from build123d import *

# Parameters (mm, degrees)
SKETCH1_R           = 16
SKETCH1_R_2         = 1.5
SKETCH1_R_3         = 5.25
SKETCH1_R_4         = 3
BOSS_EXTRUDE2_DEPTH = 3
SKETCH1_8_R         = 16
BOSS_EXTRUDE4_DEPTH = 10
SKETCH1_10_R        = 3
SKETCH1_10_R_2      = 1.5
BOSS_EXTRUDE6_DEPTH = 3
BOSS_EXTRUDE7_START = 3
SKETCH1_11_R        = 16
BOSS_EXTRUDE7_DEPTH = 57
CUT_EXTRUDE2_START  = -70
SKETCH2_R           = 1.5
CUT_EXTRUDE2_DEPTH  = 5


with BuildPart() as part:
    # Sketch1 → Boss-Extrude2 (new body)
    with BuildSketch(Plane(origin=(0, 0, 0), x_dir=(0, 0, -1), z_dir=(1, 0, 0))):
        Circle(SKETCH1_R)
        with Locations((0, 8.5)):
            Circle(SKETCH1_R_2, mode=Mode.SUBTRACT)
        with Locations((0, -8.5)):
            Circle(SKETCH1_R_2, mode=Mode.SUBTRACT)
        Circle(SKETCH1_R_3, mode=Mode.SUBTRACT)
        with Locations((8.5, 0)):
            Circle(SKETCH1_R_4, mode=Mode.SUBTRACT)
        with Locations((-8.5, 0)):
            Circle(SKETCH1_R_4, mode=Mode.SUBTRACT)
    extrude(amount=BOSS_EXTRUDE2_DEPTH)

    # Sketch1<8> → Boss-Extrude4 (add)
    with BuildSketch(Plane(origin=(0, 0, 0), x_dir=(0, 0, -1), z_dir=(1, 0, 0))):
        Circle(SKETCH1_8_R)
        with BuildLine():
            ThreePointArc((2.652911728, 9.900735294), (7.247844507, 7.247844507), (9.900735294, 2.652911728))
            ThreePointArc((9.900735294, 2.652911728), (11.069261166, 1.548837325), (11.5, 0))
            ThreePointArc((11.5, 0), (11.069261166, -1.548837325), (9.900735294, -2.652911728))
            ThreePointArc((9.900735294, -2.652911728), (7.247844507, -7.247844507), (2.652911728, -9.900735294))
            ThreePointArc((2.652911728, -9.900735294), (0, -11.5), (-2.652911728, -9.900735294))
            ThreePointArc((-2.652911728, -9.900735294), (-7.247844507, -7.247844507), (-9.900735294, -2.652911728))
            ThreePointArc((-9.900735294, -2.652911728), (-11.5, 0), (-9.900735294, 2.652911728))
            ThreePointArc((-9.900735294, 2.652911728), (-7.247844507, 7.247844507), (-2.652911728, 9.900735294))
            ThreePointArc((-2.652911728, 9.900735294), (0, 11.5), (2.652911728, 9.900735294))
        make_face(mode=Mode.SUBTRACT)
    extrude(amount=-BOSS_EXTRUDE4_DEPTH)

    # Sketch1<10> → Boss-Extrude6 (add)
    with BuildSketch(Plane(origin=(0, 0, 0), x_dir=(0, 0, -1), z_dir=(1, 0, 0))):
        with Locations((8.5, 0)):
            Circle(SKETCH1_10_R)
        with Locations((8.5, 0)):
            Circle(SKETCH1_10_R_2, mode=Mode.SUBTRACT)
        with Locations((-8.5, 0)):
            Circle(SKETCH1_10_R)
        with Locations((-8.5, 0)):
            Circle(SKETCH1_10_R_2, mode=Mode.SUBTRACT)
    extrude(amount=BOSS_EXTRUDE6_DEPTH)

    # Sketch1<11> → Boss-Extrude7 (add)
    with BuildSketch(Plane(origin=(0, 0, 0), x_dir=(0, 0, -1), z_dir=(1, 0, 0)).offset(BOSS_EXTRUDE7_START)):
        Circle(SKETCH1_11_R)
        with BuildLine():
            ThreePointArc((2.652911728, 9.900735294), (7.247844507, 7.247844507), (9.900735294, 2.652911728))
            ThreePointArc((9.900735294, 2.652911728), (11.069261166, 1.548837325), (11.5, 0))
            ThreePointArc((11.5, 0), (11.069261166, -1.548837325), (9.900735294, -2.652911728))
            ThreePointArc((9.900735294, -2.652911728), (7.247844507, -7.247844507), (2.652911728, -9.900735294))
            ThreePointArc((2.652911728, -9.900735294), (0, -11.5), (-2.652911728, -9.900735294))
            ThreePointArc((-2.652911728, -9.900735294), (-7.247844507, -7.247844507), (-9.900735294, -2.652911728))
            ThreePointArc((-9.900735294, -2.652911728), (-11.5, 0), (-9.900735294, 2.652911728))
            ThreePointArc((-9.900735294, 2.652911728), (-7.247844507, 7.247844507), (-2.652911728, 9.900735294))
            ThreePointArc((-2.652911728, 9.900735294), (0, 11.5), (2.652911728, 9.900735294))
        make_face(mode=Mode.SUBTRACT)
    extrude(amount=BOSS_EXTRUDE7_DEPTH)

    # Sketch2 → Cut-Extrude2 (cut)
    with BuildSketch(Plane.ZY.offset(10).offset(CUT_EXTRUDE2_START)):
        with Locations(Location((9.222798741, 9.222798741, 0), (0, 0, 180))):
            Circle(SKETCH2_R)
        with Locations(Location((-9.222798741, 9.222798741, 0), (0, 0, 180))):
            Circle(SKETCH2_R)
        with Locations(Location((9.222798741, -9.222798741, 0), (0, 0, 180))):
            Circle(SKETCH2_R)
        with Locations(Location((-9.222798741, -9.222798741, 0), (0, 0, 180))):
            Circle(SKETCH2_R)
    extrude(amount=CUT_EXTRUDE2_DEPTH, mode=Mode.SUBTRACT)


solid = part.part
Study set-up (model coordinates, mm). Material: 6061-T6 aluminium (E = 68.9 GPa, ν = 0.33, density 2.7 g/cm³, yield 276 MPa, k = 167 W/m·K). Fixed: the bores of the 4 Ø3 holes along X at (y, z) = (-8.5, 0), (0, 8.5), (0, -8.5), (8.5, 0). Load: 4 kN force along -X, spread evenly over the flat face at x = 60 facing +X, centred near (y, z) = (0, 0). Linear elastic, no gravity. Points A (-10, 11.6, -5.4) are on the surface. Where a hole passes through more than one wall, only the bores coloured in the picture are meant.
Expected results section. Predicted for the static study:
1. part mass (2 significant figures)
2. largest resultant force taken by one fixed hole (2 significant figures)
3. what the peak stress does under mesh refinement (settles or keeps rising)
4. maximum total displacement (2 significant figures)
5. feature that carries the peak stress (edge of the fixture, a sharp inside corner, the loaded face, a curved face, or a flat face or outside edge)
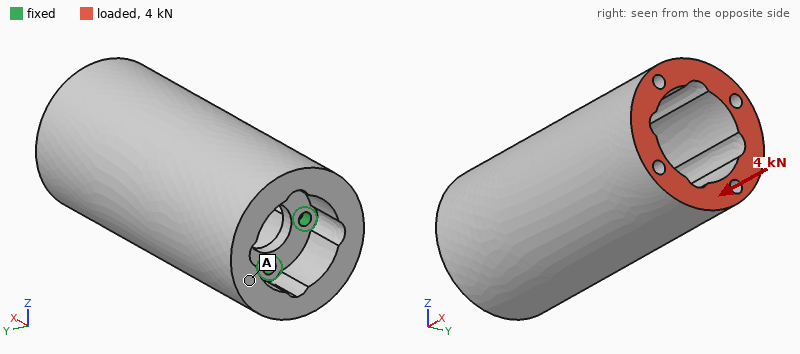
88 g
1.0 kN
keeps rising
13 µm
edge of the fixture
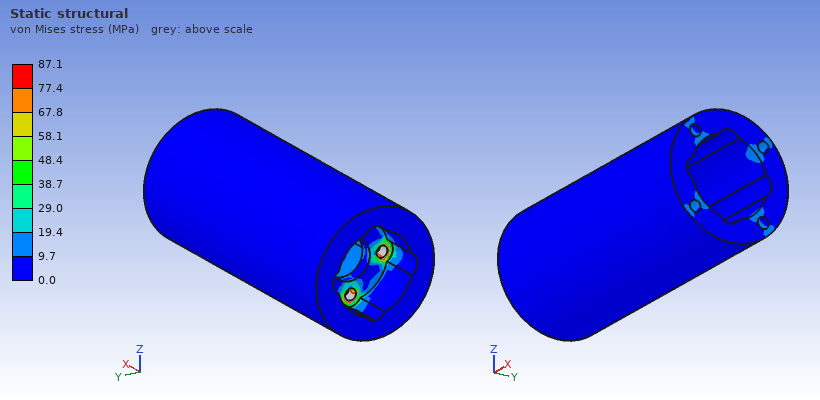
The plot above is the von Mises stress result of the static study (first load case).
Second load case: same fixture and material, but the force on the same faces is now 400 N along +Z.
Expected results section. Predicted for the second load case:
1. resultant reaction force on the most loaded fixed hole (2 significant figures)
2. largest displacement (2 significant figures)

1.1 kN
48 µm
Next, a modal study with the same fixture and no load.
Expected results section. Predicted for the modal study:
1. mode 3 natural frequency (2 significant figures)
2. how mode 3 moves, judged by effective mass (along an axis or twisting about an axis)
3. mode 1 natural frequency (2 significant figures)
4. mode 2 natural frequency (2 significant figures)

11 kHz
twisting about X
3000 Hz
3000 Hz
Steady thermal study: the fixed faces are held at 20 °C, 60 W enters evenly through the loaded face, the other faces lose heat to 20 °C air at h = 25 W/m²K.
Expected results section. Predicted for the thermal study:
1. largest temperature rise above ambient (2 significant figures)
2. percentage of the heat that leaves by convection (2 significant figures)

49 K
12 %
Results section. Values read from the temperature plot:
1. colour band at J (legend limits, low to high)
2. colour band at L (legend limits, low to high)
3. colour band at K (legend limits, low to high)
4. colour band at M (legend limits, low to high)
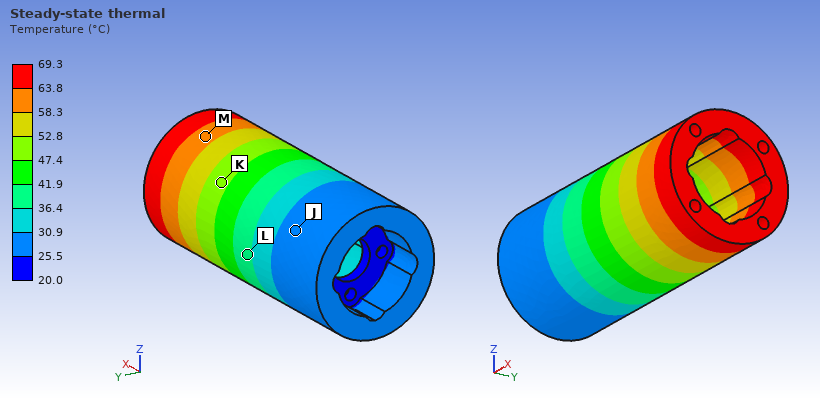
25.5 to 30.9 °C
36.4 to 41.9 °C
47.4 to 52.8 °C
58.3 to 63.8 °C
